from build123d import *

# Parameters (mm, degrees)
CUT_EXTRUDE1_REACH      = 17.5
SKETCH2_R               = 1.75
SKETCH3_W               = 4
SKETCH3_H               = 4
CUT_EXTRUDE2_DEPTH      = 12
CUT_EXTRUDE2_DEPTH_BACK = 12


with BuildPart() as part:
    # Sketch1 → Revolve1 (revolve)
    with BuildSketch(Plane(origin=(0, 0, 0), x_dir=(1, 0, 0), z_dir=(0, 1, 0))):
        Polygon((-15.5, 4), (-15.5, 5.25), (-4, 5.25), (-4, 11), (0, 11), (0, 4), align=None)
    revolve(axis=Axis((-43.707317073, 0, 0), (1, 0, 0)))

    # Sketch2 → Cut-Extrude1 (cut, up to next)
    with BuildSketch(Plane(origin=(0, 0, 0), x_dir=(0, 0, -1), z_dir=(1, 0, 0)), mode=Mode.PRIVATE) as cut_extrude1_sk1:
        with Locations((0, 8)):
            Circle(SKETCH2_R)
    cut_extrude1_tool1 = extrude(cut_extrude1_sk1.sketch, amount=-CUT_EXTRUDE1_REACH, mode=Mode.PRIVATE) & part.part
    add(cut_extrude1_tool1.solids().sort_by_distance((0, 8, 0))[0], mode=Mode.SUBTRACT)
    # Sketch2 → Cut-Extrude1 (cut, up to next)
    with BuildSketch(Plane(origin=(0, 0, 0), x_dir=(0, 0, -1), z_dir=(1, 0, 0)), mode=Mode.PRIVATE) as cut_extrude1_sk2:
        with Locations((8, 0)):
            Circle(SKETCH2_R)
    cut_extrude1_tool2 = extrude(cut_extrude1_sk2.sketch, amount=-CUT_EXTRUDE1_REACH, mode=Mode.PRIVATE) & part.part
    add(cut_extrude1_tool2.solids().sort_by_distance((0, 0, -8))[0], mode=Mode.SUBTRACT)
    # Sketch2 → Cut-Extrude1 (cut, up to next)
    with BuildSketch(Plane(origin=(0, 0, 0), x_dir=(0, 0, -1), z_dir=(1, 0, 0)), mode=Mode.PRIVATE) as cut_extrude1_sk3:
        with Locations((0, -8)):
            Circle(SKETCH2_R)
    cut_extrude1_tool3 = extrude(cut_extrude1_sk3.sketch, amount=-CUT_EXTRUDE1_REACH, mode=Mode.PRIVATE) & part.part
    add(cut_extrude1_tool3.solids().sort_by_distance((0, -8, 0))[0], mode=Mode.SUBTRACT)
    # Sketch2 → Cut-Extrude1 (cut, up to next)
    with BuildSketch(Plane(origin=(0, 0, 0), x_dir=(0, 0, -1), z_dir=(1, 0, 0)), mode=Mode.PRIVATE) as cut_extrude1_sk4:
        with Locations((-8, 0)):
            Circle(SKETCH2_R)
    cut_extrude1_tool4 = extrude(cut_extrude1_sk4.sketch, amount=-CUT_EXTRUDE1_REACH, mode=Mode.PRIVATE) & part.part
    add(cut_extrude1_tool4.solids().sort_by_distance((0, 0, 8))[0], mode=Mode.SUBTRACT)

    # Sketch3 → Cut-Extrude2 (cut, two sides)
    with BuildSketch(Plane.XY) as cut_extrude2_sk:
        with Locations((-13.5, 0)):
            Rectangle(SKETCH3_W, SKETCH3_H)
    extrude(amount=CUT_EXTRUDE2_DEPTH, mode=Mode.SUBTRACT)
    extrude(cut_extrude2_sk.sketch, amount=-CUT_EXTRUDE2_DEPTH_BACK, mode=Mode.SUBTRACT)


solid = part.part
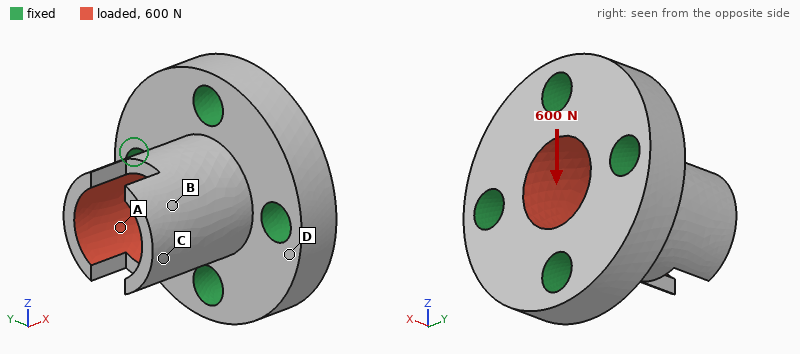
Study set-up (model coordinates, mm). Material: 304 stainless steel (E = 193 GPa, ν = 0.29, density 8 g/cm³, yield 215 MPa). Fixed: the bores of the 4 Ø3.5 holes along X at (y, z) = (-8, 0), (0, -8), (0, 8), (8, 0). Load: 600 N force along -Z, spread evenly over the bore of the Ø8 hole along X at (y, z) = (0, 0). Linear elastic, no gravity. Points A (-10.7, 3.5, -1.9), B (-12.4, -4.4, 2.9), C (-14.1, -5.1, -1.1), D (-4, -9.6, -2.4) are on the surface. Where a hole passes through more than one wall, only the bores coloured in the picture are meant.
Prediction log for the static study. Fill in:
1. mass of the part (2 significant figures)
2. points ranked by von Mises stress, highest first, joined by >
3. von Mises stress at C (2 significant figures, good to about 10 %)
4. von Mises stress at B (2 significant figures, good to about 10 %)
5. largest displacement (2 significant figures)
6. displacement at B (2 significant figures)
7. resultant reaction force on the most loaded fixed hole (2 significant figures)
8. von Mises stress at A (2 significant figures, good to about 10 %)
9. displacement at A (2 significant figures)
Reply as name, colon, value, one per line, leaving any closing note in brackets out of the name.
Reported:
mass of the part: 12 g
points ranked by von Mises stress, highest first, joined by >: A > B > C > D
von Mises stress at C: 8.6 MPa
von Mises stress at B: 12 MPa
largest displacement: 5.5 µm
displacement at B: 3.3 µm
resultant reaction force on the most loaded fixed hole: 280 N
von Mises stress at A: 22 MPa
displacement at A: 2.7 µm
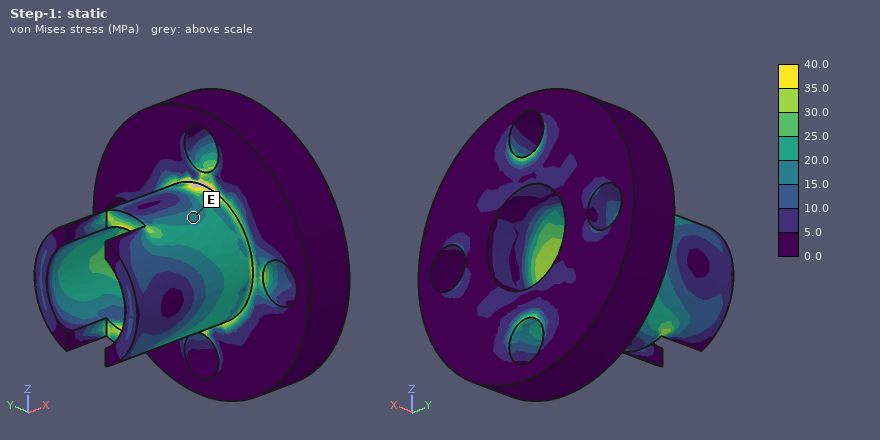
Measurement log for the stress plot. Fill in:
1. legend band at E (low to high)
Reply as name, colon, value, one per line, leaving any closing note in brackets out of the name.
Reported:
legend band at E: 15.0 to 20.0 MPa
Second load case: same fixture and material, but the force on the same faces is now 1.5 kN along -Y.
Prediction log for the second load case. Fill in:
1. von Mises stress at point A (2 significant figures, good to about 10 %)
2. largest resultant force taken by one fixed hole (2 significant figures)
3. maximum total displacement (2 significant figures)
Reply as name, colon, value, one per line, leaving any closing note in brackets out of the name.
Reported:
von Mises stress at point A: 34 MPa
largest resultant force taken by one fixed hole: 690 N
maximum total displacement: 13 µm
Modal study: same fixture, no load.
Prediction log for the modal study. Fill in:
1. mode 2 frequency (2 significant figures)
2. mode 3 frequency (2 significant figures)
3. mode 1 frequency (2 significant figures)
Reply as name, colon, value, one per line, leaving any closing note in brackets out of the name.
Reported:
mode 2 frequency: 33 kHz
mode 3 frequency: 34 kHz
mode 1 frequency: 31 kHz
